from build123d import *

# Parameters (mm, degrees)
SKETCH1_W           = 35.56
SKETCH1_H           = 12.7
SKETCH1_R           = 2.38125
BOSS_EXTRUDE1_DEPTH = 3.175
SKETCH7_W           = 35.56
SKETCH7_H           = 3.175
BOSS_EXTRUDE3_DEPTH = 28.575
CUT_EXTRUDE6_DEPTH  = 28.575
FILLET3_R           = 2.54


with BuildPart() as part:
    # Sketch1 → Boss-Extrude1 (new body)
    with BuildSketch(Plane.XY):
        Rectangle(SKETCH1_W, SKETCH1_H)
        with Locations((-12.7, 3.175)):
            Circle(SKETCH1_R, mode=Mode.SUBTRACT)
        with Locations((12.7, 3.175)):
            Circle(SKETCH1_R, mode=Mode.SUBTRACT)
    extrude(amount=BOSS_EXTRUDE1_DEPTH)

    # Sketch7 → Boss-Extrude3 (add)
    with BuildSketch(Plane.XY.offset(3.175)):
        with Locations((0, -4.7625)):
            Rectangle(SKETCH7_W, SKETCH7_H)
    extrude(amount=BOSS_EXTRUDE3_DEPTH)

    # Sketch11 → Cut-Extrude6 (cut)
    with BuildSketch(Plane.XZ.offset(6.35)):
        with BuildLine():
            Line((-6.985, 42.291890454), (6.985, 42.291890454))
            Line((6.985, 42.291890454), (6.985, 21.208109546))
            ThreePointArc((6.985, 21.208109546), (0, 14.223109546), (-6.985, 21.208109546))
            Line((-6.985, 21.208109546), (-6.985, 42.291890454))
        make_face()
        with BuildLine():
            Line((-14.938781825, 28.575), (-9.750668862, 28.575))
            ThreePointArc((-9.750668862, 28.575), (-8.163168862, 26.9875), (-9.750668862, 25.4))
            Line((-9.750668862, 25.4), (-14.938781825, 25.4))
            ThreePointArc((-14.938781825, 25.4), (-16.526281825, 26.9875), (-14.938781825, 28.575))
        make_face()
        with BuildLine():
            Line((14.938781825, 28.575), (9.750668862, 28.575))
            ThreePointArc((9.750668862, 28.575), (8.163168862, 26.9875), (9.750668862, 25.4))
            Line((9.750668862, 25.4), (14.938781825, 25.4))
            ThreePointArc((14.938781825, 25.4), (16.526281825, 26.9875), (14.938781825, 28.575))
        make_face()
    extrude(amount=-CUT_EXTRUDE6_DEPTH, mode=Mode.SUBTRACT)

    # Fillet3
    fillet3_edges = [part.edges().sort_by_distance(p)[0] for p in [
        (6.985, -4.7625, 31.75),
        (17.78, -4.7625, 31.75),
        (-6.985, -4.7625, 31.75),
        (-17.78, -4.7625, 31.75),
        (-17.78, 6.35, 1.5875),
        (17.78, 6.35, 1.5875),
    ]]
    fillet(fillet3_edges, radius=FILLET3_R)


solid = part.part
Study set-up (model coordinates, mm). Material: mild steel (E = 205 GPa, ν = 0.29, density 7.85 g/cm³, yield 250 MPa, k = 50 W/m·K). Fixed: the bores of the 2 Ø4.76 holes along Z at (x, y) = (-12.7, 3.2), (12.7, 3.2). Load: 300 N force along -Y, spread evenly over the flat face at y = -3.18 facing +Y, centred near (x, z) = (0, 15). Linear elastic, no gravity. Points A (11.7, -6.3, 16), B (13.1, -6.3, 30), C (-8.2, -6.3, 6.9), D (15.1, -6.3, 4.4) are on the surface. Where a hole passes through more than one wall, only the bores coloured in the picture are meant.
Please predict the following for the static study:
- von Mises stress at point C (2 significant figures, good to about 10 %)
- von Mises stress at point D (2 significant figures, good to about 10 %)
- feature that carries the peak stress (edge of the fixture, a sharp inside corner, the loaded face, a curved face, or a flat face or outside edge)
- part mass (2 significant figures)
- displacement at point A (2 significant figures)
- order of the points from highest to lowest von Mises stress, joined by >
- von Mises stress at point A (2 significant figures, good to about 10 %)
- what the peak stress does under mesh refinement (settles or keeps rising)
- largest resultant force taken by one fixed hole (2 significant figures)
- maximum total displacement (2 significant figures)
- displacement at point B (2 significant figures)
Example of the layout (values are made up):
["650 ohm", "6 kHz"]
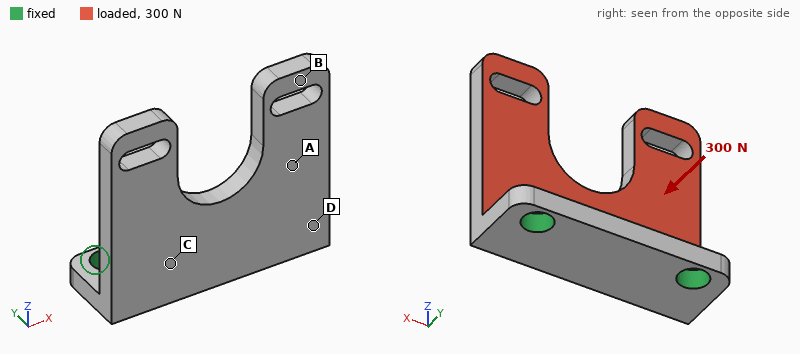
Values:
["38 MPa", "51 MPa", "edge of the fixture", "29 g", "35 µm", "D > C > A > B", "19 MPa", "keeps rising", "150 N", "86 µm", "79 µm"]
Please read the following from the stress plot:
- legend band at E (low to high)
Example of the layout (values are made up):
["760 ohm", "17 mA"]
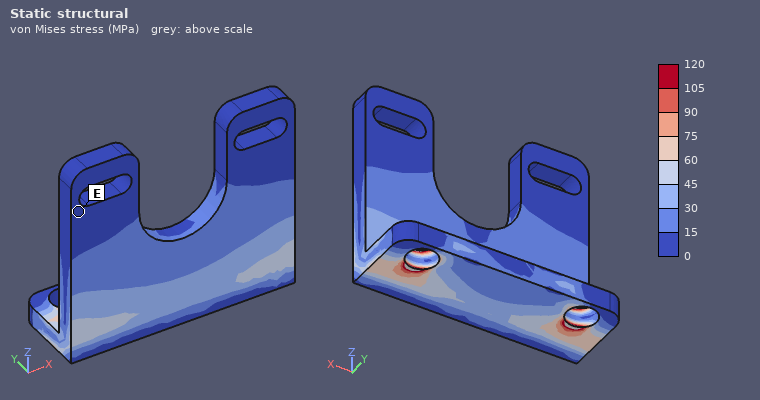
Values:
["0 to 15 MPa"]
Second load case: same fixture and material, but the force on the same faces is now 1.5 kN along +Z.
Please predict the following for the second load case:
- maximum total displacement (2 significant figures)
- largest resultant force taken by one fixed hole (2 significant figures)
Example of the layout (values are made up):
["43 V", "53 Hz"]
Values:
["14 µm", "750 N"]
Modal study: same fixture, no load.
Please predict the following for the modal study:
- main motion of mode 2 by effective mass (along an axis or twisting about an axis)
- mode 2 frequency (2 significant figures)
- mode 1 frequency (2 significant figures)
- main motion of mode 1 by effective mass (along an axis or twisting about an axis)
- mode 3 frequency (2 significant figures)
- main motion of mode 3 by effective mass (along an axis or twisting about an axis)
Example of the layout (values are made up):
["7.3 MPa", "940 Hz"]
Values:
["twisting about Z", "4100 Hz", "2900 Hz", "along Y", "9700 Hz", "along X"]
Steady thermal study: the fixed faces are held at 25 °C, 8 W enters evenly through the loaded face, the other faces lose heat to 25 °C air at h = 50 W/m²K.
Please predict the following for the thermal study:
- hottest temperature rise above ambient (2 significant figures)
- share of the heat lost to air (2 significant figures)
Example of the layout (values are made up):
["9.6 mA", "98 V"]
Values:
["28 K", "20 %"]
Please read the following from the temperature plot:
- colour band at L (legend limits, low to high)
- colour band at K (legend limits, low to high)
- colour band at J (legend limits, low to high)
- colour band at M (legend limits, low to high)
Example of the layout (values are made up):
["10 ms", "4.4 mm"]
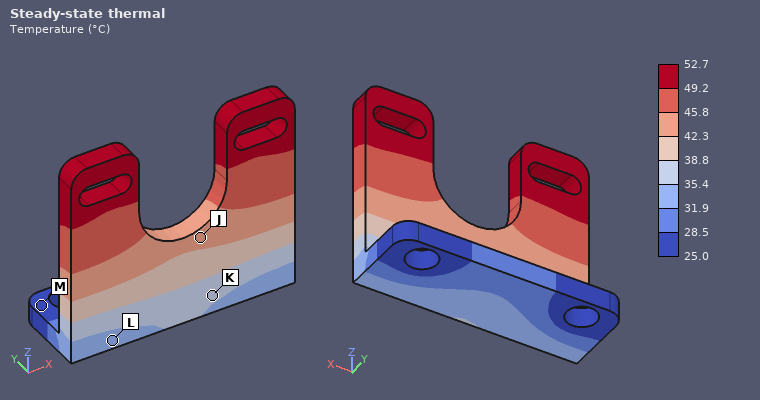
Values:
["31.9 to 35.4 °C", "35.4 to 38.8 °C", "42.3 to 45.8 °C", "25.0 to 28.5 °C"]
